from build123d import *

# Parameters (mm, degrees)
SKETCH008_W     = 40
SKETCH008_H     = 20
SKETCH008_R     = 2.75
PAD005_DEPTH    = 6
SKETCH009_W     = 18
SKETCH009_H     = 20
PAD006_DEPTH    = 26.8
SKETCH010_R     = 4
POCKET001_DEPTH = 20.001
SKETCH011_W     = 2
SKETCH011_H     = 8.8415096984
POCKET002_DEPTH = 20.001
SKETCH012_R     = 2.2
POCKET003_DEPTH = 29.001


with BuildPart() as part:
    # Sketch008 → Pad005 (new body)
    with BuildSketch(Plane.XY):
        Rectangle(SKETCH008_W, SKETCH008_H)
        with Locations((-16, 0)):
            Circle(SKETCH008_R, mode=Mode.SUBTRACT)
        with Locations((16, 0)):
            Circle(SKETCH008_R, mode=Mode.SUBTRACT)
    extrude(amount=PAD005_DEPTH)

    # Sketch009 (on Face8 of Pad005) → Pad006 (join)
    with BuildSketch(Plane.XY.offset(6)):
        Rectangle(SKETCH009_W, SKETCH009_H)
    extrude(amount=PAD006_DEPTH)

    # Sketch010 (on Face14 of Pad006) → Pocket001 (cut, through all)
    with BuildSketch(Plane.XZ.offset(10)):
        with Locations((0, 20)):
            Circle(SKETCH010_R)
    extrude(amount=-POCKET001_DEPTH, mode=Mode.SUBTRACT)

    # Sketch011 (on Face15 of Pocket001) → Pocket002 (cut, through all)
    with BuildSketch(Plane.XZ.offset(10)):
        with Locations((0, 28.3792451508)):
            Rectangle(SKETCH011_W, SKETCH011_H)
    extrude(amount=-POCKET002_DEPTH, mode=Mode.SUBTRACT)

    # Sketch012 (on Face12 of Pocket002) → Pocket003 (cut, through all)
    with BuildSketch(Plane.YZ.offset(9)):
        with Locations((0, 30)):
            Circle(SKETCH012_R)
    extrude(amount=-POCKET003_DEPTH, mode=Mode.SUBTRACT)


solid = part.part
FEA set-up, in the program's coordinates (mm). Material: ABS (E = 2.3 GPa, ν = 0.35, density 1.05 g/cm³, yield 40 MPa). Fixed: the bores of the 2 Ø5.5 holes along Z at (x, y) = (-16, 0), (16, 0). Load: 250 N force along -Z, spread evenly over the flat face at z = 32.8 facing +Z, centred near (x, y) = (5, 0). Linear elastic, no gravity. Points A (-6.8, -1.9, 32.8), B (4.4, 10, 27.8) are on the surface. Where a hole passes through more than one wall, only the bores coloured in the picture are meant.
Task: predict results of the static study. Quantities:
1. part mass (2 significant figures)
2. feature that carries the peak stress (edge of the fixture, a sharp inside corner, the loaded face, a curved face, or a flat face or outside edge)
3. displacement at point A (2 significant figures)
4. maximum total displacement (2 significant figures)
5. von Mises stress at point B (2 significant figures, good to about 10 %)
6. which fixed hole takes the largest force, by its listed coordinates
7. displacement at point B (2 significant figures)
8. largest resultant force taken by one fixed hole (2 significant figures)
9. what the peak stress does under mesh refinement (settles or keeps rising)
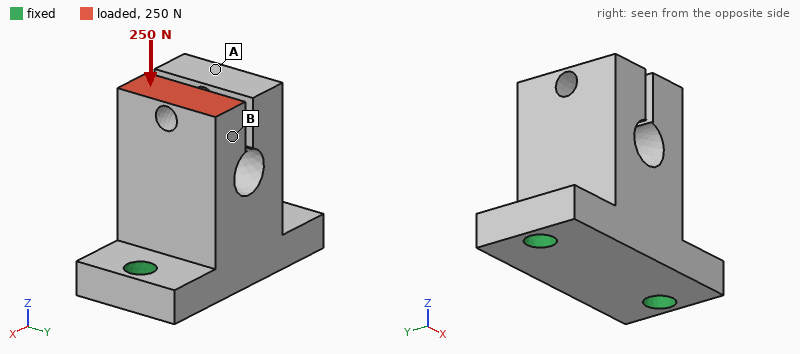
13 g
edge of the fixture
35 µm
89 µm
1.8 MPa
(16, 0)
54 µm
180 N
keeps rising
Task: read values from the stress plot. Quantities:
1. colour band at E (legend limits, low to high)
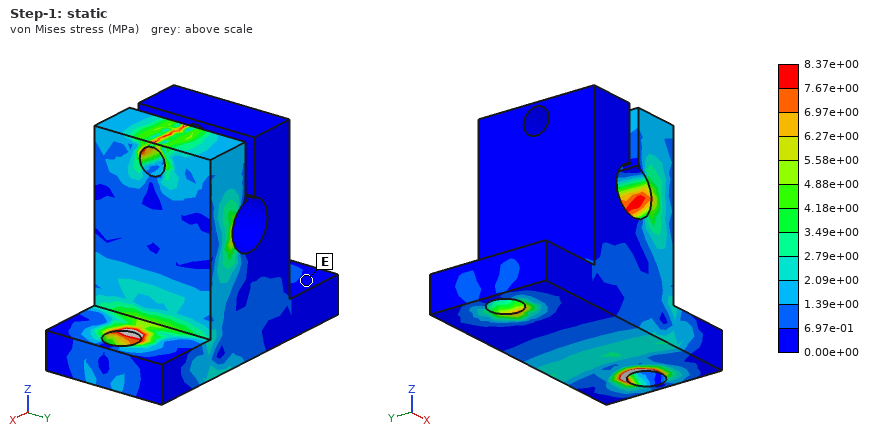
0.00e+00 to 6.97e-01 MPa
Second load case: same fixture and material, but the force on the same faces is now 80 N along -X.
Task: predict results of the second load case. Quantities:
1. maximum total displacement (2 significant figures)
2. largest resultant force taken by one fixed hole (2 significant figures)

0.35 mm
110 N
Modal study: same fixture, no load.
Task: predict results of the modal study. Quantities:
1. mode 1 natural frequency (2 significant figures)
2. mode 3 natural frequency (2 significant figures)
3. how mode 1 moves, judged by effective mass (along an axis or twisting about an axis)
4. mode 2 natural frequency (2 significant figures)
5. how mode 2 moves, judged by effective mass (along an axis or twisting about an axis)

1500 Hz
3100 Hz
along Y
2400 Hz
along X
